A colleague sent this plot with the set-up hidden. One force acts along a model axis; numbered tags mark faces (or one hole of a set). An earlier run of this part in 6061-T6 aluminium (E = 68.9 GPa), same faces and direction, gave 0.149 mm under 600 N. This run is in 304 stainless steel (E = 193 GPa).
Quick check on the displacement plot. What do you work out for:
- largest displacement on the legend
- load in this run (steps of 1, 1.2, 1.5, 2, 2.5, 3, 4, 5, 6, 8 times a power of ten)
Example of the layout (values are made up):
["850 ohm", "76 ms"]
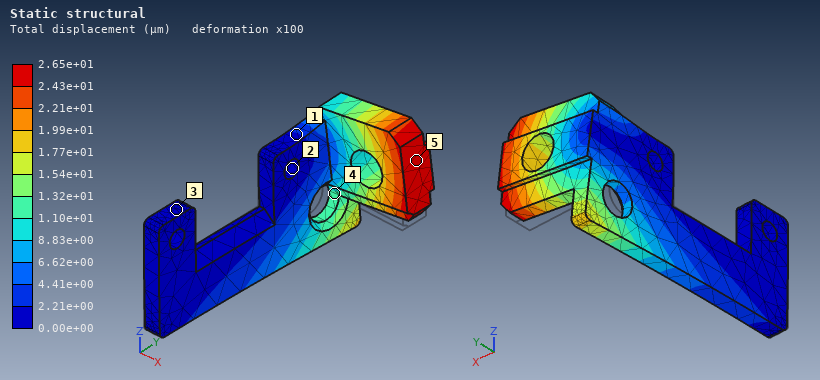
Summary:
["2.65e+01 µm", "300 N"]
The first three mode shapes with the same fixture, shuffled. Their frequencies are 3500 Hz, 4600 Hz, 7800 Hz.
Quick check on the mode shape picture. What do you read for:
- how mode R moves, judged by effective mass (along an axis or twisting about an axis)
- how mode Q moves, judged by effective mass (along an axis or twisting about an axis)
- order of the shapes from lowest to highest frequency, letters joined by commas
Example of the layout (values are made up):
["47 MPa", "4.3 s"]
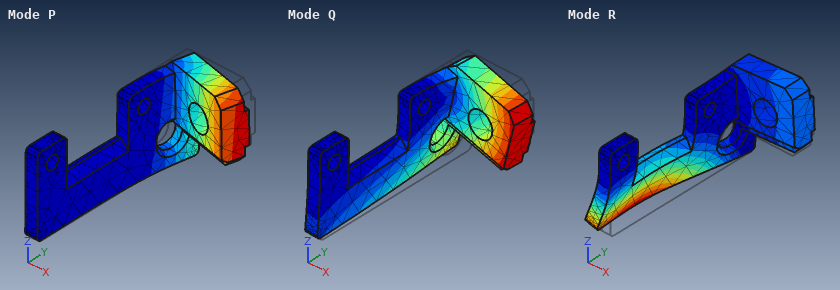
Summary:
["along X", "along Z", "P, Q, R"]
